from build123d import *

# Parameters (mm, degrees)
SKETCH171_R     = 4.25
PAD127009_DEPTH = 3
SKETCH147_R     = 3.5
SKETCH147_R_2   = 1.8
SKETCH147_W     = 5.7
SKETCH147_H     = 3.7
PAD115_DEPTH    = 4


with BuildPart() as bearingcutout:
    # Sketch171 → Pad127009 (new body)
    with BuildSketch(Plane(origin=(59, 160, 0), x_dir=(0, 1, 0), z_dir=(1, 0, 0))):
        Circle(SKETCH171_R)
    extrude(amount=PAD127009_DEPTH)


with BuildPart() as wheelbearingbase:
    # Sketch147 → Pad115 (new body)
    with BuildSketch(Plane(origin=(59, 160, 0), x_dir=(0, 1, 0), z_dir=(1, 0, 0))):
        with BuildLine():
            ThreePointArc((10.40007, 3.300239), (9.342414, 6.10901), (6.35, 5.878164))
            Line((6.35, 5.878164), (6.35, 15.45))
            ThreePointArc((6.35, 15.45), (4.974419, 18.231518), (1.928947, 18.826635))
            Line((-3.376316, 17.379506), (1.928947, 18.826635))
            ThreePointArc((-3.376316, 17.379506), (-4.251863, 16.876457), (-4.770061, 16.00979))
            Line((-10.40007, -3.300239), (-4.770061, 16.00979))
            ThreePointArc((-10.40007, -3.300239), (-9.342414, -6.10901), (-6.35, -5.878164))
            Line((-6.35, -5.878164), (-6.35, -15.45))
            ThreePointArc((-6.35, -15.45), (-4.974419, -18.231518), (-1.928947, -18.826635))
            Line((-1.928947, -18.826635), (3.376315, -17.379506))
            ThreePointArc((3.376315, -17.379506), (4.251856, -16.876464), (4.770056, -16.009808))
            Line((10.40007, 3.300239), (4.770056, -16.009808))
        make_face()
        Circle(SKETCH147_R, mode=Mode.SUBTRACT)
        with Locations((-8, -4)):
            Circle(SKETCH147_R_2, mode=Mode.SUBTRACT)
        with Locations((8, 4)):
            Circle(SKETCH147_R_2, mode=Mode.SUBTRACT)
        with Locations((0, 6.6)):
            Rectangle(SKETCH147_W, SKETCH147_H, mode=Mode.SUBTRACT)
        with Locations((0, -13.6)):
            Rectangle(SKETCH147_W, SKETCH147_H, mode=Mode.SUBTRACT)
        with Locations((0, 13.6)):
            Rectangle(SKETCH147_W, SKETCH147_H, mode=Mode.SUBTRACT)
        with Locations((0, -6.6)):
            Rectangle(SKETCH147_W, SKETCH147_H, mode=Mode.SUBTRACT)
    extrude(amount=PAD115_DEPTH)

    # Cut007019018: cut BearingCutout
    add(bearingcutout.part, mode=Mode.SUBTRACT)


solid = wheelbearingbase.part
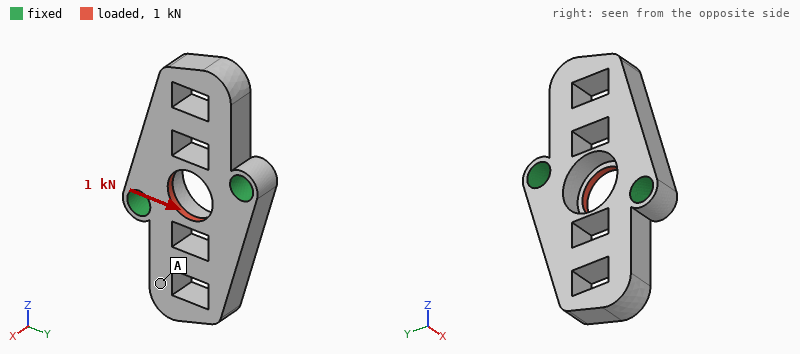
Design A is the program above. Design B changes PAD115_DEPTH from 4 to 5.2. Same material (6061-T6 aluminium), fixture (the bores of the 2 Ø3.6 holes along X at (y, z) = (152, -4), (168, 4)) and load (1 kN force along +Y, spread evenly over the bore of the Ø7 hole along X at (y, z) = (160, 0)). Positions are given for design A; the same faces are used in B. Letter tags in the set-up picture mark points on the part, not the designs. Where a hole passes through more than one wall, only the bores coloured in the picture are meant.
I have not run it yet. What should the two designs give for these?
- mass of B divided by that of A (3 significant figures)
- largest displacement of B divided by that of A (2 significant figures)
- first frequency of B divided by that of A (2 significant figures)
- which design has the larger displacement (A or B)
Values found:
1.31
0.64
1.2
A
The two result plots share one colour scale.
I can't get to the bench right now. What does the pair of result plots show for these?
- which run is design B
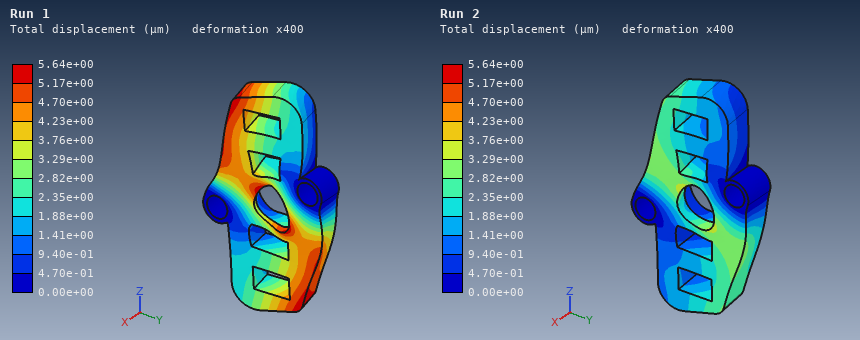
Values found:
Run 2
